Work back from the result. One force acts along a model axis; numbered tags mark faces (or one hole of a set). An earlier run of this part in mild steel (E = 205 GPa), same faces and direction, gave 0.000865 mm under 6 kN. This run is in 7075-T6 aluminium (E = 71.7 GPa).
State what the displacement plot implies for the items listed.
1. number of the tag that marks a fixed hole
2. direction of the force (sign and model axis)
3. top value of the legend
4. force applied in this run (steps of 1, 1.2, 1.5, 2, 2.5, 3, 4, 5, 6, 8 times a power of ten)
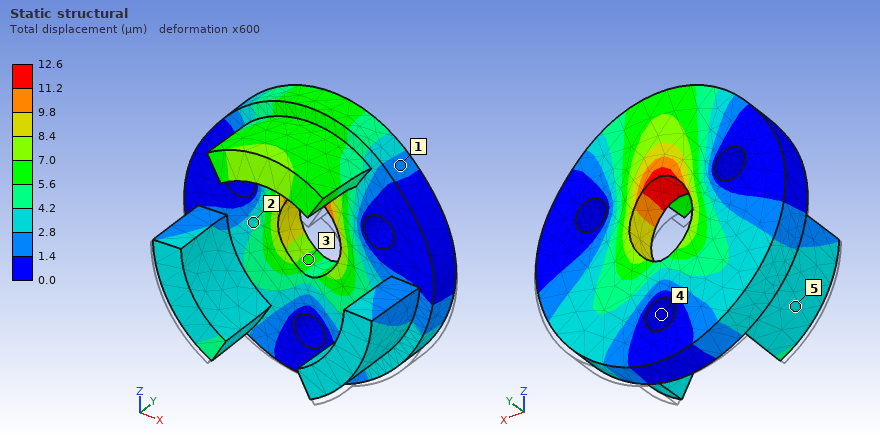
4
+Z
12.6 µm
30 kN
